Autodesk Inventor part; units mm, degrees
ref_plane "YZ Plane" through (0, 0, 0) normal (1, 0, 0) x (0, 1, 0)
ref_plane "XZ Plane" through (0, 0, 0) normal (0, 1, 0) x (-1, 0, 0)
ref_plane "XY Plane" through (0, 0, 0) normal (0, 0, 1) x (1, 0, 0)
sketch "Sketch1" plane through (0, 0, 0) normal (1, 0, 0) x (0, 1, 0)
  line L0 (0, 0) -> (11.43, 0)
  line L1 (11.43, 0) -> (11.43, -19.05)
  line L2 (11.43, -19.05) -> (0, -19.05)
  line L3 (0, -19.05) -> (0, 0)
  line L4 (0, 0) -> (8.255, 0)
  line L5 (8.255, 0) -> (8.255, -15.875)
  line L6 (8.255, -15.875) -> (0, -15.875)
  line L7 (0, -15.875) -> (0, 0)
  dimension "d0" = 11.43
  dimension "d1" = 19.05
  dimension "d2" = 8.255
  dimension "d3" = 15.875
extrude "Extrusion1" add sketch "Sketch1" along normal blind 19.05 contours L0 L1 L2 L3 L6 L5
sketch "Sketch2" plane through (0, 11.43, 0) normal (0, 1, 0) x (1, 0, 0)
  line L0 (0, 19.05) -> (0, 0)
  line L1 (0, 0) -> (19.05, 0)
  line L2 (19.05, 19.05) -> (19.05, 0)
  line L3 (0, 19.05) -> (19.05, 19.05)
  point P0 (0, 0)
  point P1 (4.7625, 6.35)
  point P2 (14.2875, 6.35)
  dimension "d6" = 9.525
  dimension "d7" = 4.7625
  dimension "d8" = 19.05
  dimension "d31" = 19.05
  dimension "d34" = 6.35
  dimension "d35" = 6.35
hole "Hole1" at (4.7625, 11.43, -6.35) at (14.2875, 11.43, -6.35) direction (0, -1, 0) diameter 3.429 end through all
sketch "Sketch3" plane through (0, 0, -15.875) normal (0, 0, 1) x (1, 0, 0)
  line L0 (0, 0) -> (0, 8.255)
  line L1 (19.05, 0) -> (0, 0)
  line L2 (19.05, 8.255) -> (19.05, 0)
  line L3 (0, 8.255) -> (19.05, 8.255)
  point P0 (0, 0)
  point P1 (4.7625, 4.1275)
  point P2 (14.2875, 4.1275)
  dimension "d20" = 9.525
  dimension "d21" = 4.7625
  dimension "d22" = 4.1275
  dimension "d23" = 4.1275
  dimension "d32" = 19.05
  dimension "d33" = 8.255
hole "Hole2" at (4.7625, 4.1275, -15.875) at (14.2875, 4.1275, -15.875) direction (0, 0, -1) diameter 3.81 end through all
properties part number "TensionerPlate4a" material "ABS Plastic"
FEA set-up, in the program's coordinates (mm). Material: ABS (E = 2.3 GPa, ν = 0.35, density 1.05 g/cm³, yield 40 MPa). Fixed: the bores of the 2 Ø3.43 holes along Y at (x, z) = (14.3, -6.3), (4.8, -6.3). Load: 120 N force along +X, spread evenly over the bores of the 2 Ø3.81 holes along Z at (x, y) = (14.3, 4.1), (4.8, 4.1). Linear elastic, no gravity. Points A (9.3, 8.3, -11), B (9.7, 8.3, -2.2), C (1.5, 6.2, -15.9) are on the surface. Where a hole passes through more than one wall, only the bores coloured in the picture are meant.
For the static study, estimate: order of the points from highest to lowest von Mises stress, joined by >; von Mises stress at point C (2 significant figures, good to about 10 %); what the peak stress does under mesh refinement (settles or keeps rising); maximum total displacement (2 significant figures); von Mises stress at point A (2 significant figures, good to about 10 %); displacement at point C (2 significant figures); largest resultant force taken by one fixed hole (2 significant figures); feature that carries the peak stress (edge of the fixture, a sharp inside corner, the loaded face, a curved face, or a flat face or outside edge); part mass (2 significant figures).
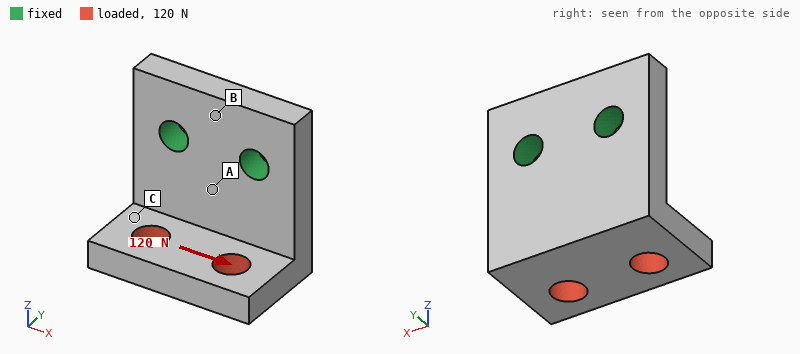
A > C > B
7.9 MPa
keeps rising
0.34 mm
15 MPa
0.20 mm
130 N
edge of the fixture
1.6 g
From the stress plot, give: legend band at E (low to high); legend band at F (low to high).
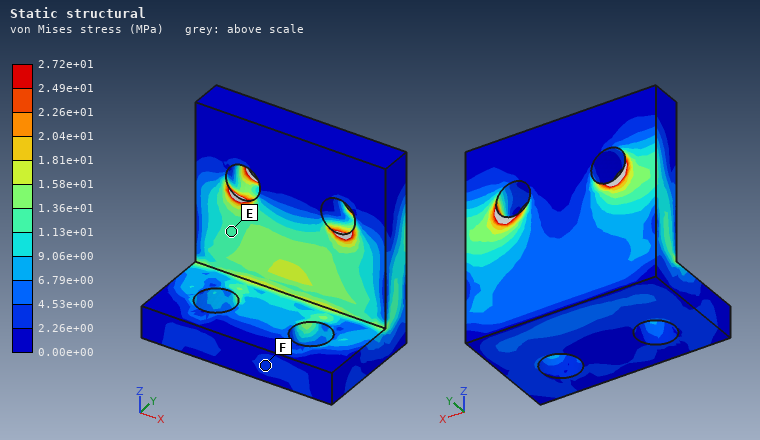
1.13e+01 to 1.36e+01 MPa
2.26e+00 to 4.53e+00 MPa
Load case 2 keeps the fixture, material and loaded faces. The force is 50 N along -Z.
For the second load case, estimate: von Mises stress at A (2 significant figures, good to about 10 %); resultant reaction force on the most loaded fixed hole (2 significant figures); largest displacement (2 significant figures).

8.4 MPa
26 N
0.32 mm
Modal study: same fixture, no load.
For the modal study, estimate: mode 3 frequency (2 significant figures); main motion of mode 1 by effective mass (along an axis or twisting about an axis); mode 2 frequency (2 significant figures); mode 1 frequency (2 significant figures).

7100 Hz
along Y
4200 Hz
2600 Hz
